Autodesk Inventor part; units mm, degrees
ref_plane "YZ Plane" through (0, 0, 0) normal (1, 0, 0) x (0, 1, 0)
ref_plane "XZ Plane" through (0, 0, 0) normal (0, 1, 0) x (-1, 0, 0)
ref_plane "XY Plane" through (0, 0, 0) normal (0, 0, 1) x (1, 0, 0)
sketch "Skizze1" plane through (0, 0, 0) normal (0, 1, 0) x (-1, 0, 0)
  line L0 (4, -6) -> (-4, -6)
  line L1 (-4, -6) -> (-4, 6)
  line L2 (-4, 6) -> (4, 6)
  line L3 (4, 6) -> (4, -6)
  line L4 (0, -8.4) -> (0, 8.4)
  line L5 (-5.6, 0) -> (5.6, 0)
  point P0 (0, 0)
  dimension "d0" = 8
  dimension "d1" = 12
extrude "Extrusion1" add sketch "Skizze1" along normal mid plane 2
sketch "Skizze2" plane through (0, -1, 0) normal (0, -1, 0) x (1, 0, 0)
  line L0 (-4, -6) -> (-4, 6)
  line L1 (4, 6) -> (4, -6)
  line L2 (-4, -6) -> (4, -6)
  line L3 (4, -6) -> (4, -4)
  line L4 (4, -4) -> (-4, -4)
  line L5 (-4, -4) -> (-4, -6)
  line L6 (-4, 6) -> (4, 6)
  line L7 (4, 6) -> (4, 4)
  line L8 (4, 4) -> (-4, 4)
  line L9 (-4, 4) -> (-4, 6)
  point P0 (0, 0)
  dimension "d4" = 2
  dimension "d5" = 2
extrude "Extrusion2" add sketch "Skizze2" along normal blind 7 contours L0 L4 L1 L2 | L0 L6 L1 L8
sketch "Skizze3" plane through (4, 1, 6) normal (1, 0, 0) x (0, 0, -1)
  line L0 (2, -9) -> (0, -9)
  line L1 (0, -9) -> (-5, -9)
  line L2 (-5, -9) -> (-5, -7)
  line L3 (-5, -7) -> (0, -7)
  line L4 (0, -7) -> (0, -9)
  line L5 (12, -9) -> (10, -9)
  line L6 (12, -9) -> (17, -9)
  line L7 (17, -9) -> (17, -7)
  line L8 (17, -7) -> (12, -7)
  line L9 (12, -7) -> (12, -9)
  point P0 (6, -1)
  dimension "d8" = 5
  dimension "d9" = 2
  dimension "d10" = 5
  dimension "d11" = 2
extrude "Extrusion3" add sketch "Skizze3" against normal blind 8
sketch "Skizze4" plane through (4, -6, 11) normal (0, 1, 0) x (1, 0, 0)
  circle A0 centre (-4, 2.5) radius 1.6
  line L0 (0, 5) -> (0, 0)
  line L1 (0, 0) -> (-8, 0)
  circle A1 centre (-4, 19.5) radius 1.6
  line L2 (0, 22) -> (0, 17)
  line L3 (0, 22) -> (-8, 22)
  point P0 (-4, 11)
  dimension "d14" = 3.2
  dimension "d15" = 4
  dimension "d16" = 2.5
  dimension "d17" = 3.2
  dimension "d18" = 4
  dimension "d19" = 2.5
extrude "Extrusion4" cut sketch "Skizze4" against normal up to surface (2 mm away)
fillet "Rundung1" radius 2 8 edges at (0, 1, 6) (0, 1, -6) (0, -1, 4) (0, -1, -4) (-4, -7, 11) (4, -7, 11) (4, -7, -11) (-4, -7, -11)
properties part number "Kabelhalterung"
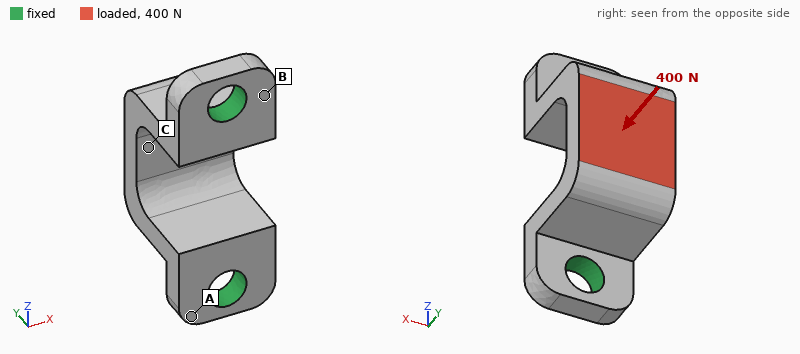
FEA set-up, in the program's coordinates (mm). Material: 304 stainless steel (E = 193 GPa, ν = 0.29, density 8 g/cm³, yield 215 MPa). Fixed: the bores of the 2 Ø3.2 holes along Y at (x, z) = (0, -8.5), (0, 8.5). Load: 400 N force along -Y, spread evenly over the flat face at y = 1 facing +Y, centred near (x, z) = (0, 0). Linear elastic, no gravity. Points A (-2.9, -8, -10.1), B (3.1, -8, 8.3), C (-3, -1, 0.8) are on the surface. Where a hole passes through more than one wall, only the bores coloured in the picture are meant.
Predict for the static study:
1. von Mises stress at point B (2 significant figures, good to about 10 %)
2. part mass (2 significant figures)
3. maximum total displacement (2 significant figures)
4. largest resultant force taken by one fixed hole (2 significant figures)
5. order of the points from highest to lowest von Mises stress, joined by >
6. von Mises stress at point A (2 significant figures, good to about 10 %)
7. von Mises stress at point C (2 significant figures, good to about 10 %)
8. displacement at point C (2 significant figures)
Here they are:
12 MPa
4.3 g
2.6 µm
220 N
C > B > A
6.8 MPa
24 MPa
2.4 µm
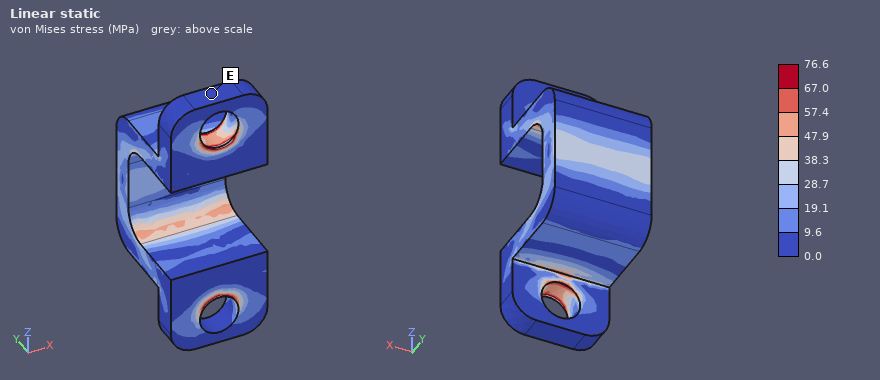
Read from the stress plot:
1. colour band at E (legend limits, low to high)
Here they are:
0.0 to 9.6 MPa
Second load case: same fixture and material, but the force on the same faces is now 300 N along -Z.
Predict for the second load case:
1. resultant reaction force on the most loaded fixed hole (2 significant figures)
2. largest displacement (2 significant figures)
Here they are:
210 N
5.4 µm
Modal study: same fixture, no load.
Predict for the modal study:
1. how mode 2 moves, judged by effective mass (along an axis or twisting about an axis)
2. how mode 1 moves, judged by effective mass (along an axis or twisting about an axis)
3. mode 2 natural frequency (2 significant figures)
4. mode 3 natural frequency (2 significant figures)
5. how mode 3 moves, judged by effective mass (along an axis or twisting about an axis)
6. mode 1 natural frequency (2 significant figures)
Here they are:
along Z
along X
26 kHz
33 kHz
twisting about Y
19 kHz
